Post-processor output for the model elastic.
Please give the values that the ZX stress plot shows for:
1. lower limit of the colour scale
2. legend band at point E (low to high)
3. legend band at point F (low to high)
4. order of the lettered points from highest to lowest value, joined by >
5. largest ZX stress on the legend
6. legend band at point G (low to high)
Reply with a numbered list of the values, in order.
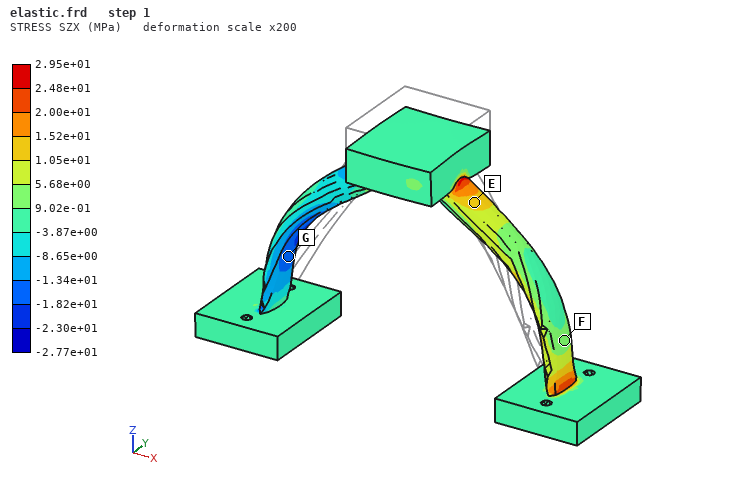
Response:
1. -2.77e+01 MPa
2. 1.05e+01 to 1.52e+01 MPa
3. 9.02e-01 to 5.68e+00 MPa
4. E > F > G
5. 2.95e+01 MPa
6. -1.82e+01 to -1.34e+01 MPa
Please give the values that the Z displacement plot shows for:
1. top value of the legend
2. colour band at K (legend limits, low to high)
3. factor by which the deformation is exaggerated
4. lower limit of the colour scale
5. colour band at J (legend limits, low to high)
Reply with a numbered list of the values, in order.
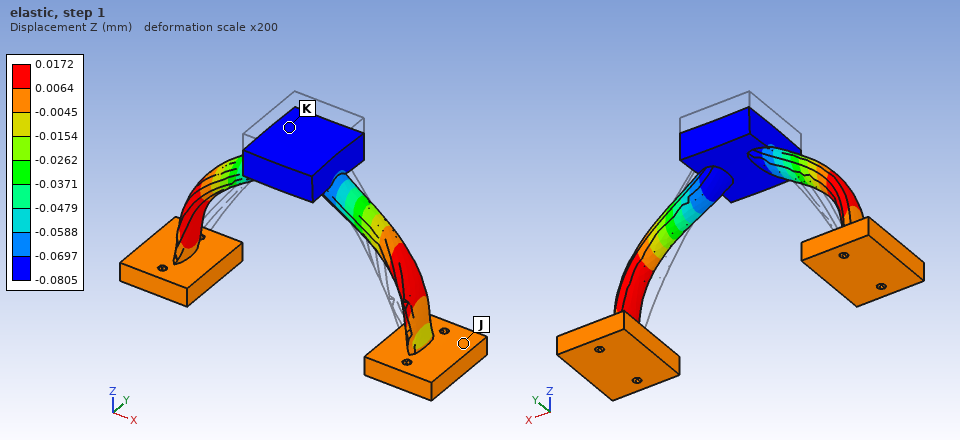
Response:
1. 0.0172 mm
2. -0.0805 to -0.0697 mm
3. 200
4. -0.0805 mm
5. -0.0045 to 0.0064 mm
